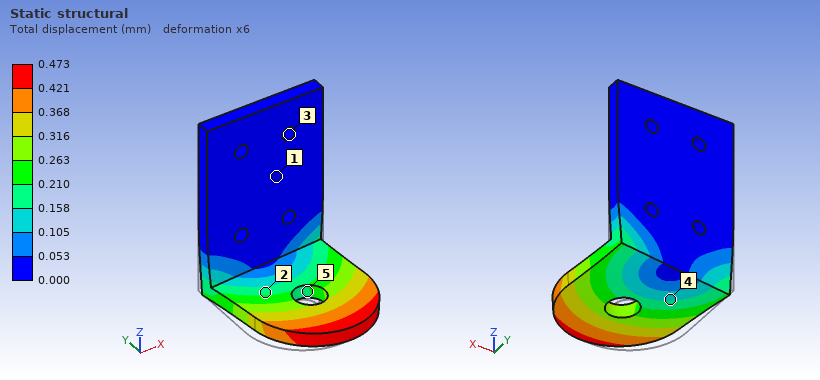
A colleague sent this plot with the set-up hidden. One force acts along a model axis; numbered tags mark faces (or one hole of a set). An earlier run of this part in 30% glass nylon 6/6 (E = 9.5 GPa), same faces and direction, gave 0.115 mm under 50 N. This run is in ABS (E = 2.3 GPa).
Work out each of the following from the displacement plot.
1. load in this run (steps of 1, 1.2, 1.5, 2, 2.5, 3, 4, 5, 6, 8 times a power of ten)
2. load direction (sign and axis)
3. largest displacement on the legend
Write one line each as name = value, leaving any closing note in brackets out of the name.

load in this run = 50 N
load direction = +X
largest displacement on the legend = 0.473 mm
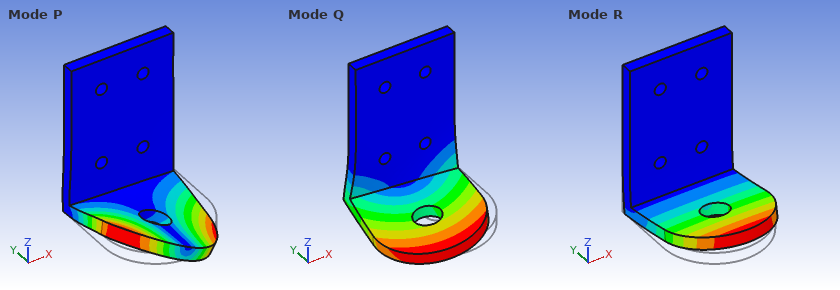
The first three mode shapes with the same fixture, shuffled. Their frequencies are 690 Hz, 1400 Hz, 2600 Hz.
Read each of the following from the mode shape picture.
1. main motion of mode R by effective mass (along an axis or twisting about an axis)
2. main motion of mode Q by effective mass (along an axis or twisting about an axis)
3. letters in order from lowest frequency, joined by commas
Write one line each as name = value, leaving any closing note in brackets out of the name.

main motion of mode R by effective mass = along Z
main motion of mode Q by effective mass = along X
letters in order from lowest frequency, joined by commas = R, Q, P
